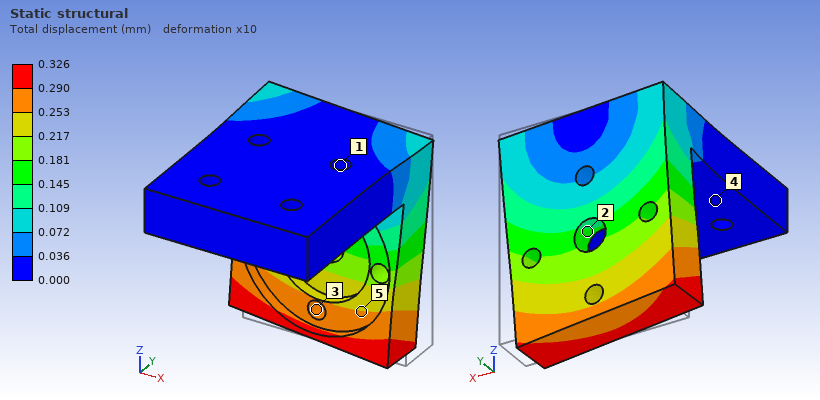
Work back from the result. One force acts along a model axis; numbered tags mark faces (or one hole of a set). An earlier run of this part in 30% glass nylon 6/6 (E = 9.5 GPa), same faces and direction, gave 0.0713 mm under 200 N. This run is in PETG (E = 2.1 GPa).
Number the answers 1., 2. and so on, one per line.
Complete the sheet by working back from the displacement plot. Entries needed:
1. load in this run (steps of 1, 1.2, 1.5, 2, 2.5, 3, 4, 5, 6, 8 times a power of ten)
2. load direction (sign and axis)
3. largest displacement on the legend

1. 200 N
2. -X
3. 0.326 mm
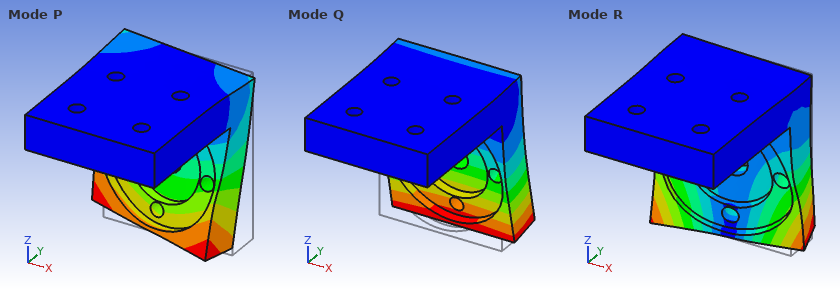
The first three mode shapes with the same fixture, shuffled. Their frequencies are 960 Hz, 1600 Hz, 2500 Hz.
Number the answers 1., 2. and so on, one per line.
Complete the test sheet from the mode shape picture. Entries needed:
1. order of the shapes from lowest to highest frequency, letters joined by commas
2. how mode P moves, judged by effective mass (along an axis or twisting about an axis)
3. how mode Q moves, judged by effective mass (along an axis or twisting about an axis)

1. Q, P, R
2. along X
3. along Y
